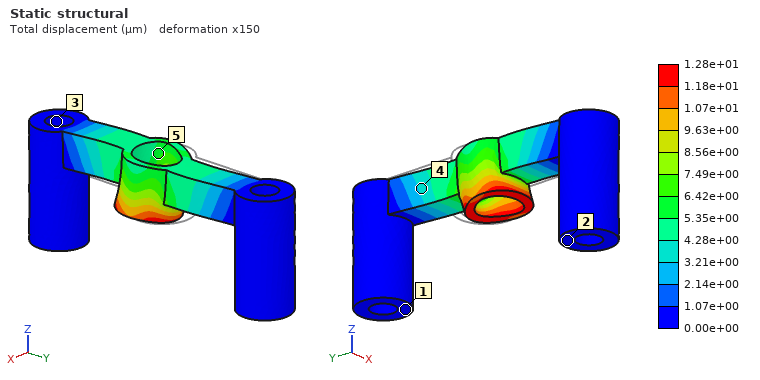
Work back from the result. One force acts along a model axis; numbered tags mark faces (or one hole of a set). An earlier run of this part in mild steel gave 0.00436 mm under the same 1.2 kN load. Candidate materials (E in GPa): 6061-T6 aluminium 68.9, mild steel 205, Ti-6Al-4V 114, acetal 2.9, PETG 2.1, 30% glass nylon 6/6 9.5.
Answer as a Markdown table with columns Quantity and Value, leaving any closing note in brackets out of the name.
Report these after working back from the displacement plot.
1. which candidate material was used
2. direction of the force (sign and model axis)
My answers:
| Quantity | Value |
|---|---|
| which candidate material was used | 6061-T6 aluminium |
| direction of the force | -Y |
